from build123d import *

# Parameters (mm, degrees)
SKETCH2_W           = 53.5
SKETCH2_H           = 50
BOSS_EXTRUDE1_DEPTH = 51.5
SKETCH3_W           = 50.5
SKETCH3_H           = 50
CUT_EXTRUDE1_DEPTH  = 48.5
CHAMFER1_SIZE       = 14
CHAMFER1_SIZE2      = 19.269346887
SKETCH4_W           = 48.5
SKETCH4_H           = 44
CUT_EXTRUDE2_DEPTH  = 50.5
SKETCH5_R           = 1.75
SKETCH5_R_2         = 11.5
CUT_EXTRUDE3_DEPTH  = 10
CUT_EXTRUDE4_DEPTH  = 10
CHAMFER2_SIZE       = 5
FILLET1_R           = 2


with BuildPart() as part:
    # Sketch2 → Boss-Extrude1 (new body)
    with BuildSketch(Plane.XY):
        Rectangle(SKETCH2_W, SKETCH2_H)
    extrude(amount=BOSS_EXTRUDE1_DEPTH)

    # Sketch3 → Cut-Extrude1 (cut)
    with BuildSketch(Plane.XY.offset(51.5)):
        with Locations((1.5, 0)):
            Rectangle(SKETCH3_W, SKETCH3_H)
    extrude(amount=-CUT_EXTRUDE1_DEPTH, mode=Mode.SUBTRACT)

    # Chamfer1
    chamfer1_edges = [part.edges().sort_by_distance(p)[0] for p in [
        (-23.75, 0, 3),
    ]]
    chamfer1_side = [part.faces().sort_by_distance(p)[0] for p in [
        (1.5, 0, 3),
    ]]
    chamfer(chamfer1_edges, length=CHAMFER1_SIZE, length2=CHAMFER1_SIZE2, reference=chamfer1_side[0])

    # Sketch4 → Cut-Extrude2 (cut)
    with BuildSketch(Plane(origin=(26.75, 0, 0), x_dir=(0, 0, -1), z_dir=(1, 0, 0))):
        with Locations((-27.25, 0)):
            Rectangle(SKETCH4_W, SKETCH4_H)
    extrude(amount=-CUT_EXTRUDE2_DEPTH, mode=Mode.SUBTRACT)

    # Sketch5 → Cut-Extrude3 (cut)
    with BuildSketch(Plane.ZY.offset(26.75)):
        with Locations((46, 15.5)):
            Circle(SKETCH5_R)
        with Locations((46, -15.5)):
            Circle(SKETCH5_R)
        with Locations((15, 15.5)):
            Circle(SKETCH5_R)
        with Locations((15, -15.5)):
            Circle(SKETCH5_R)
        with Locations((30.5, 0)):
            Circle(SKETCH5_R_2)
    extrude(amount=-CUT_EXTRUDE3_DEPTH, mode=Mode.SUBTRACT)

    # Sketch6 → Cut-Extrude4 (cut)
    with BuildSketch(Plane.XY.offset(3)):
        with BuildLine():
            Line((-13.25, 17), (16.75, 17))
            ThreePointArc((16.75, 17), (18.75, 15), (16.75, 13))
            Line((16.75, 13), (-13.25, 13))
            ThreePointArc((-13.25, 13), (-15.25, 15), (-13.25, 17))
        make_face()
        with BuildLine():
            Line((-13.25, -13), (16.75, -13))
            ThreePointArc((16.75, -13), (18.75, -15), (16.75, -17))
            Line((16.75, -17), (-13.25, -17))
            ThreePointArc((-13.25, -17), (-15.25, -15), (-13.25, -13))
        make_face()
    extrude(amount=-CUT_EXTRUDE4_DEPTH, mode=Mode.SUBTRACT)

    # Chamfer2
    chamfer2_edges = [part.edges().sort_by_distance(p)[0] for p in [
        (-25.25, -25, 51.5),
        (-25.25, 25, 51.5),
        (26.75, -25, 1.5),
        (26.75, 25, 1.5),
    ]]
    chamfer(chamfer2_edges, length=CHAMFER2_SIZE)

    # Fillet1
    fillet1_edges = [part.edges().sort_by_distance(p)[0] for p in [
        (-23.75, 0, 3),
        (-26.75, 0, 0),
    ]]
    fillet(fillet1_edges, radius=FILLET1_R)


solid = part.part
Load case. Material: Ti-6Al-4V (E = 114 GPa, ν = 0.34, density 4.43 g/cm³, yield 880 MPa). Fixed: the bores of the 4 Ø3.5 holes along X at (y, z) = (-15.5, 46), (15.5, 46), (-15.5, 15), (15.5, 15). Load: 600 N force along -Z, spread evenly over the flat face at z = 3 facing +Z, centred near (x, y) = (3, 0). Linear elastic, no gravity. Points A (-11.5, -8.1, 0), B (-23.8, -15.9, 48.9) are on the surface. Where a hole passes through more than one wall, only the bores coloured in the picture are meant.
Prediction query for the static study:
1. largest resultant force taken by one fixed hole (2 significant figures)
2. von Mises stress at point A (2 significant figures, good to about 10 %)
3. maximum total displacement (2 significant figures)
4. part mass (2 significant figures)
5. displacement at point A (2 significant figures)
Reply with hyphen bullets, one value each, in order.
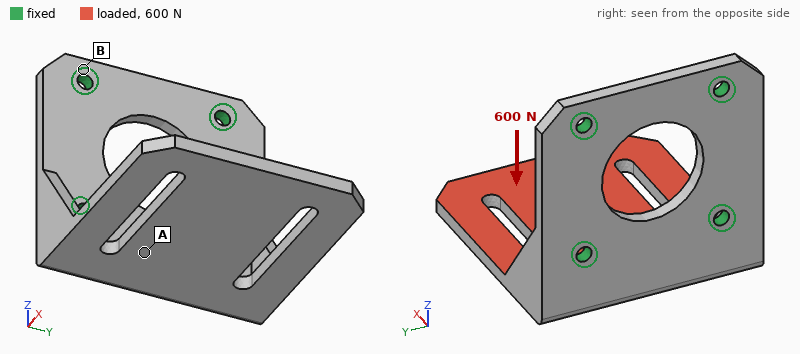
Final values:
- 320 N
- 96 MPa
- 0.92 mm
- 61 g
- 0.17 mm
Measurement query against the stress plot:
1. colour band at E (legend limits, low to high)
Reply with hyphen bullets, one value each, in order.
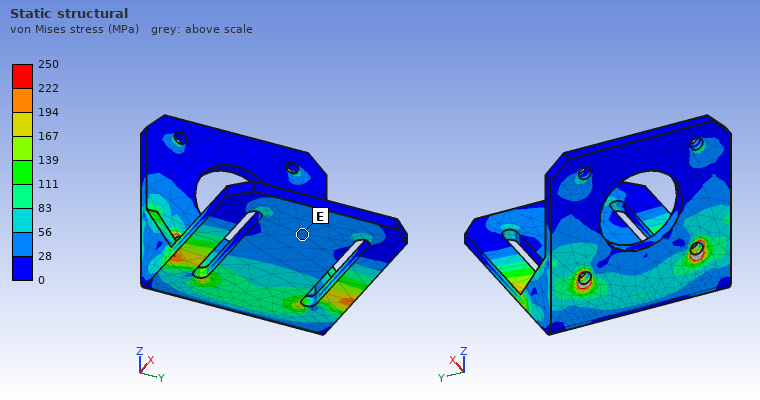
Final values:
- 28 to 56 MPa
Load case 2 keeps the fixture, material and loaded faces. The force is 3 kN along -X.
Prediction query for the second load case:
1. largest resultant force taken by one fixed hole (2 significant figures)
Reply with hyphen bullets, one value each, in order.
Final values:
- 1.7 kN
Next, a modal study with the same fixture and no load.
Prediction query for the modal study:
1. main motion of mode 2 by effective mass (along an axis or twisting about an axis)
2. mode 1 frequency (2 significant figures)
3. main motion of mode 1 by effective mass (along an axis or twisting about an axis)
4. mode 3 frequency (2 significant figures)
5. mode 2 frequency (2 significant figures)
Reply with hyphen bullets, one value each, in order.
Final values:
- along Y
- 960 Hz
- along Z
- 3300 Hz
- 2100 Hz
